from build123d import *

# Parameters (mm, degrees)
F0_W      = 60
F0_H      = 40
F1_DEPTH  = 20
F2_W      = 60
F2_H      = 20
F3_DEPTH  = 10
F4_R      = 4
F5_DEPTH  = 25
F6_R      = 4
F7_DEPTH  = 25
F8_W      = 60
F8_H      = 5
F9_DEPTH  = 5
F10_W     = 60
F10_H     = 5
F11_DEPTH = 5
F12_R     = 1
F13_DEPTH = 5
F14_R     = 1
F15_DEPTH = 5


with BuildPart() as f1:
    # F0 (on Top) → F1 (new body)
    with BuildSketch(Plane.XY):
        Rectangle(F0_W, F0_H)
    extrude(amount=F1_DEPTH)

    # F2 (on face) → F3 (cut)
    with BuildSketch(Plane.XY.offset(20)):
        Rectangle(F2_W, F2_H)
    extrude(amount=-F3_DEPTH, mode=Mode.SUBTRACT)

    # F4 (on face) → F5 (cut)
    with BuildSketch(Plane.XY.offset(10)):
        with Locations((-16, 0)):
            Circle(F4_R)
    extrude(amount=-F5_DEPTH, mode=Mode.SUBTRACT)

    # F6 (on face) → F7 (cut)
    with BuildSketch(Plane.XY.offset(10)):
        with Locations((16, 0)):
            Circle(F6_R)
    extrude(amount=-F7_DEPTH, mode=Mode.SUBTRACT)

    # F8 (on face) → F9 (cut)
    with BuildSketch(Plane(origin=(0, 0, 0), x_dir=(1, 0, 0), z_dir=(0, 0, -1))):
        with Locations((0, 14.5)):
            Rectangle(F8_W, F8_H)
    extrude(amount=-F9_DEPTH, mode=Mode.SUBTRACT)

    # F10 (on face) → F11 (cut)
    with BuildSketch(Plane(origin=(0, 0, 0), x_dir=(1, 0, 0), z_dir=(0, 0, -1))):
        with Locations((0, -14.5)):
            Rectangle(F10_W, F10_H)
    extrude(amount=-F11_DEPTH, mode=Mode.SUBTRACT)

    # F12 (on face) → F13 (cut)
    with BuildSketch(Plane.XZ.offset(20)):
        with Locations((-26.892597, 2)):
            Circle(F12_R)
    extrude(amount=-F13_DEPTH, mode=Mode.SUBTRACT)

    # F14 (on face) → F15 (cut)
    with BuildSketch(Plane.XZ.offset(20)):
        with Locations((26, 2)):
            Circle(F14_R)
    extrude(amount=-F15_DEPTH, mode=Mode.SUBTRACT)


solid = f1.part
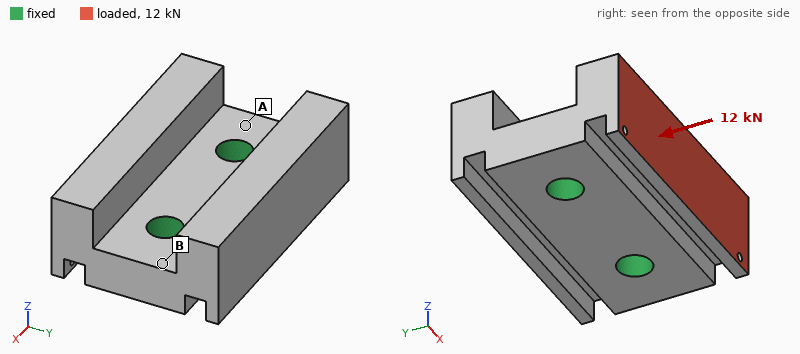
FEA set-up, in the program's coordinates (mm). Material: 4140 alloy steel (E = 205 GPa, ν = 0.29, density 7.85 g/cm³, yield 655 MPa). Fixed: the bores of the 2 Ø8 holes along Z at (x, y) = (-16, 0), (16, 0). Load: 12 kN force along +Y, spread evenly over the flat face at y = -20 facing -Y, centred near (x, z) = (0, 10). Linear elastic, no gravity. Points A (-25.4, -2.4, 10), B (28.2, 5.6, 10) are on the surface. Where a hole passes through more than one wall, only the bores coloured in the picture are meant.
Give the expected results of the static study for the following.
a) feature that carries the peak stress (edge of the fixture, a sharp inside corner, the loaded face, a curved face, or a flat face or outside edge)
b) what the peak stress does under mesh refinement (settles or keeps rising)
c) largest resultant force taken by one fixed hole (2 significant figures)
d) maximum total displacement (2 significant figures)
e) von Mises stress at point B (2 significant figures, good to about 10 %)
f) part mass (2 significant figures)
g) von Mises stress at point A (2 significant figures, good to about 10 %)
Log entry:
edge of the fixture
keeps rising
6.0 kN
23 µm
15 MPa
250 g
45 MPa
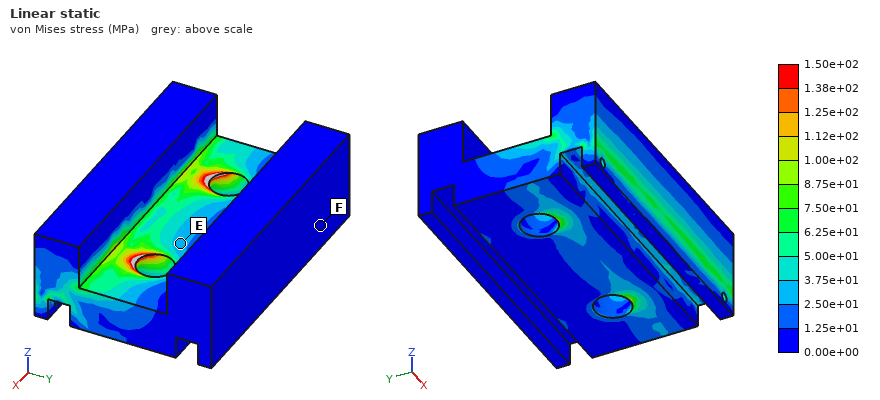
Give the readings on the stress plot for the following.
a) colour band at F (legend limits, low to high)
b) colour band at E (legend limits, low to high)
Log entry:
0.00e+00 to 1.25e+01 MPa
2.50e+01 to 3.75e+01 MPa
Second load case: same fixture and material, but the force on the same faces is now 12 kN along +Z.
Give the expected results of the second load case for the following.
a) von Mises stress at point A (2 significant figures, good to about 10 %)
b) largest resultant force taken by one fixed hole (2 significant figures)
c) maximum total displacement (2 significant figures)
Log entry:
100 MPa
6.0 kN
74 µm
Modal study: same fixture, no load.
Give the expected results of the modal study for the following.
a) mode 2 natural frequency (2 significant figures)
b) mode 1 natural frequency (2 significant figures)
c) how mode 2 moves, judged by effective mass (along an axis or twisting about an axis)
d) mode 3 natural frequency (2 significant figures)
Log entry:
11 kHz
9500 Hz
along Z
13 kHz
